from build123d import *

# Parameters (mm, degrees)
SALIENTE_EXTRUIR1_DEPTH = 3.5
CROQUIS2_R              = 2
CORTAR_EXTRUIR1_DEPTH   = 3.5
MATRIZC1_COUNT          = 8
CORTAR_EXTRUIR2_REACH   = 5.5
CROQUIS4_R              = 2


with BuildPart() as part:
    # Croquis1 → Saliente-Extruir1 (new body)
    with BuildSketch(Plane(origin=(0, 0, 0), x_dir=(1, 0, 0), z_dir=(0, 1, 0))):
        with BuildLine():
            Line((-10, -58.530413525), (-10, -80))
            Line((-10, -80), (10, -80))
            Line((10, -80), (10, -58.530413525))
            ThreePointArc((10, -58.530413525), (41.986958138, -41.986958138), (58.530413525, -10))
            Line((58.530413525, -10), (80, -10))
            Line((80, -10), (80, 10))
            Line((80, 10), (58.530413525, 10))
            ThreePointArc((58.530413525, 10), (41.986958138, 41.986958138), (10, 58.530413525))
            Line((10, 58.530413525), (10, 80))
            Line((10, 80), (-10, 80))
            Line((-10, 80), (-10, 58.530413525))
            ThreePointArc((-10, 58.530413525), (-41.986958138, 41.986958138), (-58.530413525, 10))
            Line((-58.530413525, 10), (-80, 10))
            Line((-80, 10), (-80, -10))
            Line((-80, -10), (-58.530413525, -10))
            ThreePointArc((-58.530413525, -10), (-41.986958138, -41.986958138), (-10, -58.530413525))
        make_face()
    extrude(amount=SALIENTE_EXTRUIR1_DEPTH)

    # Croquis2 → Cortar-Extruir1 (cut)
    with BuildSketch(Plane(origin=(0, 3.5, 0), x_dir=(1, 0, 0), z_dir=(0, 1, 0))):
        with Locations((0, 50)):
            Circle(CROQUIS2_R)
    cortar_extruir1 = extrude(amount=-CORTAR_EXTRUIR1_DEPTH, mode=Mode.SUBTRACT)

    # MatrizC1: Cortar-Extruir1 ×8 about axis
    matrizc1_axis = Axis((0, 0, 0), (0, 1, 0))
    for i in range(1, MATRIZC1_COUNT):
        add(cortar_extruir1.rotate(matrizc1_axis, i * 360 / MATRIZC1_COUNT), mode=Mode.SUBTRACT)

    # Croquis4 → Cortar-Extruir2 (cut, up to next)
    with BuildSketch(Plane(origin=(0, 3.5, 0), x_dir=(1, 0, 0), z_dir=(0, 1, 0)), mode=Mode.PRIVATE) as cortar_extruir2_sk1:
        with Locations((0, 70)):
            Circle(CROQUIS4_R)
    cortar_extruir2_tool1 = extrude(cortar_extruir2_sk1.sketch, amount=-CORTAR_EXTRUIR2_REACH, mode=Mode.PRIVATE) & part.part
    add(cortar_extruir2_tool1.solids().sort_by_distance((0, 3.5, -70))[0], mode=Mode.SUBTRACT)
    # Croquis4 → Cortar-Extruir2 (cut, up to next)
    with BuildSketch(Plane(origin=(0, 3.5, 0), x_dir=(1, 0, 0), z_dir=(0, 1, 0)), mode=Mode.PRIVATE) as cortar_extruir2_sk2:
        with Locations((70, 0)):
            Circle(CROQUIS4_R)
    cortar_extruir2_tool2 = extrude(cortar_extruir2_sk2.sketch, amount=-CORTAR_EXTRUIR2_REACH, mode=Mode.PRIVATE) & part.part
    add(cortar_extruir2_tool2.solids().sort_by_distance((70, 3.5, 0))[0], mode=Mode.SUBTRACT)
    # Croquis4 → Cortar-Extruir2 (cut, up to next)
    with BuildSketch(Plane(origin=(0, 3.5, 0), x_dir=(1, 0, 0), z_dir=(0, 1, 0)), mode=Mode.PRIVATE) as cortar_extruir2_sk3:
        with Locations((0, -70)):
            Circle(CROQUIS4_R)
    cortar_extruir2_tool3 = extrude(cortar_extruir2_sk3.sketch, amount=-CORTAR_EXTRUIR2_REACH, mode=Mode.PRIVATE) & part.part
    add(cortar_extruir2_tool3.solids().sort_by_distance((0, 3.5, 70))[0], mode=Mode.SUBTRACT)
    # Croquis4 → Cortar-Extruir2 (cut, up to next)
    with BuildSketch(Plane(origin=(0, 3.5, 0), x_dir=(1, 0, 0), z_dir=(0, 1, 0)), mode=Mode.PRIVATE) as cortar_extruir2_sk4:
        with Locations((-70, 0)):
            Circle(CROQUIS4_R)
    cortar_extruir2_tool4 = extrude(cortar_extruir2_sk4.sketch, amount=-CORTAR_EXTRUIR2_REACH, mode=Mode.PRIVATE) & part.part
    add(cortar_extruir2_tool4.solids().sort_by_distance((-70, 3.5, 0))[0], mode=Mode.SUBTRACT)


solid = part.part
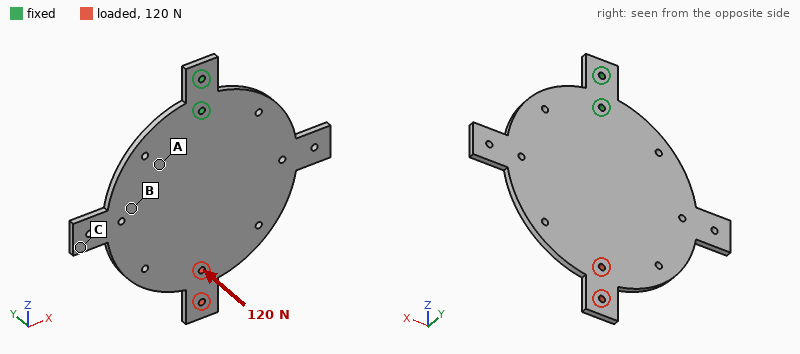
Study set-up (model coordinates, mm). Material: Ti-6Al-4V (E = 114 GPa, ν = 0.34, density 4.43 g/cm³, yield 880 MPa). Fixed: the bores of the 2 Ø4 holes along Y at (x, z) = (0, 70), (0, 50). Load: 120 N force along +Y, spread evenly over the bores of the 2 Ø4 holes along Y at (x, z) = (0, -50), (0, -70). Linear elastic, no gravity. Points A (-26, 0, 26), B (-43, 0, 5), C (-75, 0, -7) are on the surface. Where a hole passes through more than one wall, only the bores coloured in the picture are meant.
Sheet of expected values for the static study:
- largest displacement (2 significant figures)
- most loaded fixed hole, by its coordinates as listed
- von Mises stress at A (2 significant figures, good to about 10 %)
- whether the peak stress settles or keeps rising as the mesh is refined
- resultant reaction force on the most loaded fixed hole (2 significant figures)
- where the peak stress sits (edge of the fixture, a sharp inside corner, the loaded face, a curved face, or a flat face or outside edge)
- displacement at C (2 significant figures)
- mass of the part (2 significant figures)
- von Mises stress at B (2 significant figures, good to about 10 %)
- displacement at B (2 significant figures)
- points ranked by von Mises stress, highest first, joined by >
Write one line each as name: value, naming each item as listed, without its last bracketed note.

largest displacement: 2.4 mm
most loaded fixed hole, by its coordinates as listed: (0, 50)
von Mises stress at A: 49 MPa
whether the peak stress settles or keeps rising as the mesh is refined: keeps rising
resultant reaction force on the most loaded fixed hole: 410 N
where the peak stress sits: edge of the fixture
displacement at C: 0.64 mm
mass of the part: 200 g
von Mises stress at B: 27 MPa
displacement at B: 0.49 mm
points ranked by von Mises stress, highest first, joined by >: A > B > C
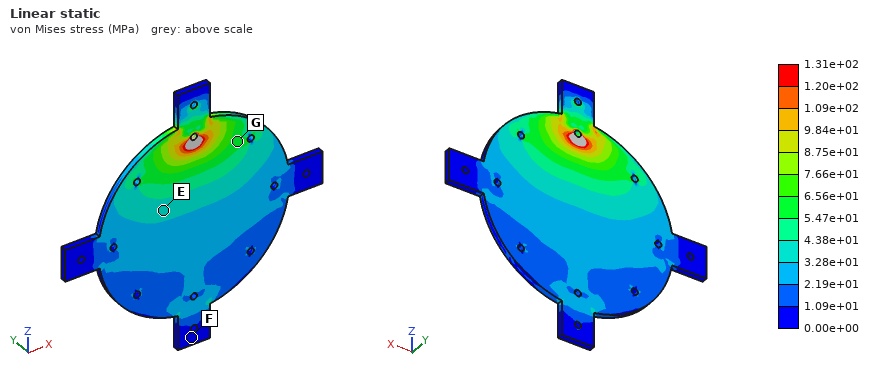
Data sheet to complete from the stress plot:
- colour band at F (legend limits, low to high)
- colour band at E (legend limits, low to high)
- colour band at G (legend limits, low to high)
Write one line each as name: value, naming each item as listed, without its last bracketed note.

colour band at F: 0.00e+00 to 1.09e+01 MPa
colour band at E: 3.28e+01 to 4.38e+01 MPa
colour band at G: 5.47e+01 to 6.56e+01 MPa
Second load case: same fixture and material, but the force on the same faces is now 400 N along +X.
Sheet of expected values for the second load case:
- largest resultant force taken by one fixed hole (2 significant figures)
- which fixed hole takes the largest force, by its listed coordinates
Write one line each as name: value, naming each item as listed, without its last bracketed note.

largest resultant force taken by one fixed hole: 2.2 kN
which fixed hole takes the largest force, by its listed coordinates: (0, 50)
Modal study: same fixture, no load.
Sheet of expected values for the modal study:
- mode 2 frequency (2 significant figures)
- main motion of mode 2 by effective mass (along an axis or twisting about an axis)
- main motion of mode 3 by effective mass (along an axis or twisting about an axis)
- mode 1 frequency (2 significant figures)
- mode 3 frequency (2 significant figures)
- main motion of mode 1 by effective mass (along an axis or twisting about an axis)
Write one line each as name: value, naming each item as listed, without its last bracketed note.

mode 2 frequency: 310 Hz
main motion of mode 2 by effective mass: twisting about Z
main motion of mode 3 by effective mass: along Y
mode 1 frequency: 190 Hz
mode 3 frequency: 750 Hz
main motion of mode 1 by effective mass: along Y
